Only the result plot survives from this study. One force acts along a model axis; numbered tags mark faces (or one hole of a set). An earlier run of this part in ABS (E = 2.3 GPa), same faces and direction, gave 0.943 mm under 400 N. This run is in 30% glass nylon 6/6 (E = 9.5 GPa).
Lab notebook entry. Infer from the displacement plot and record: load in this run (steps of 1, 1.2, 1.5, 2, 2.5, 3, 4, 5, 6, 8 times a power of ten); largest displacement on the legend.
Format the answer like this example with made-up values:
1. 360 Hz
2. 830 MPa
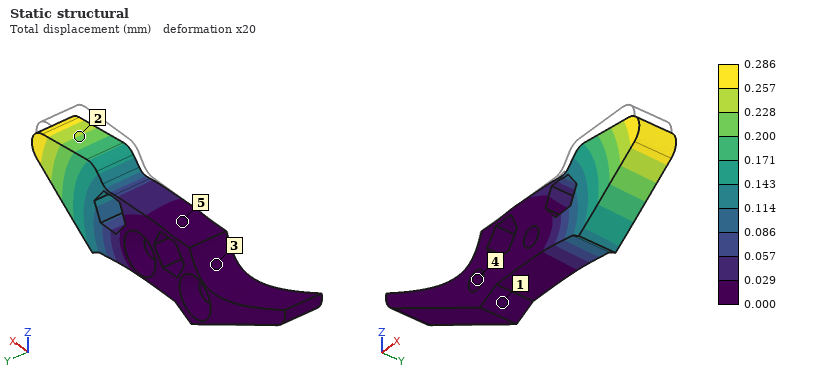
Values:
1. 500 N
2. 0.286 mm
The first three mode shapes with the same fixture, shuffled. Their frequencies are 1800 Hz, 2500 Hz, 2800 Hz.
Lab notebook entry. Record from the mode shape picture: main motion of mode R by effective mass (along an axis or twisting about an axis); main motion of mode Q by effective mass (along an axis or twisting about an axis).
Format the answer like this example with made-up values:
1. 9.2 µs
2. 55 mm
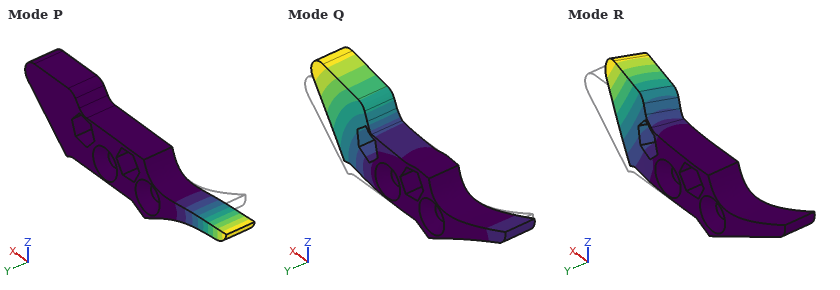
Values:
1. along Y
2. along Z
